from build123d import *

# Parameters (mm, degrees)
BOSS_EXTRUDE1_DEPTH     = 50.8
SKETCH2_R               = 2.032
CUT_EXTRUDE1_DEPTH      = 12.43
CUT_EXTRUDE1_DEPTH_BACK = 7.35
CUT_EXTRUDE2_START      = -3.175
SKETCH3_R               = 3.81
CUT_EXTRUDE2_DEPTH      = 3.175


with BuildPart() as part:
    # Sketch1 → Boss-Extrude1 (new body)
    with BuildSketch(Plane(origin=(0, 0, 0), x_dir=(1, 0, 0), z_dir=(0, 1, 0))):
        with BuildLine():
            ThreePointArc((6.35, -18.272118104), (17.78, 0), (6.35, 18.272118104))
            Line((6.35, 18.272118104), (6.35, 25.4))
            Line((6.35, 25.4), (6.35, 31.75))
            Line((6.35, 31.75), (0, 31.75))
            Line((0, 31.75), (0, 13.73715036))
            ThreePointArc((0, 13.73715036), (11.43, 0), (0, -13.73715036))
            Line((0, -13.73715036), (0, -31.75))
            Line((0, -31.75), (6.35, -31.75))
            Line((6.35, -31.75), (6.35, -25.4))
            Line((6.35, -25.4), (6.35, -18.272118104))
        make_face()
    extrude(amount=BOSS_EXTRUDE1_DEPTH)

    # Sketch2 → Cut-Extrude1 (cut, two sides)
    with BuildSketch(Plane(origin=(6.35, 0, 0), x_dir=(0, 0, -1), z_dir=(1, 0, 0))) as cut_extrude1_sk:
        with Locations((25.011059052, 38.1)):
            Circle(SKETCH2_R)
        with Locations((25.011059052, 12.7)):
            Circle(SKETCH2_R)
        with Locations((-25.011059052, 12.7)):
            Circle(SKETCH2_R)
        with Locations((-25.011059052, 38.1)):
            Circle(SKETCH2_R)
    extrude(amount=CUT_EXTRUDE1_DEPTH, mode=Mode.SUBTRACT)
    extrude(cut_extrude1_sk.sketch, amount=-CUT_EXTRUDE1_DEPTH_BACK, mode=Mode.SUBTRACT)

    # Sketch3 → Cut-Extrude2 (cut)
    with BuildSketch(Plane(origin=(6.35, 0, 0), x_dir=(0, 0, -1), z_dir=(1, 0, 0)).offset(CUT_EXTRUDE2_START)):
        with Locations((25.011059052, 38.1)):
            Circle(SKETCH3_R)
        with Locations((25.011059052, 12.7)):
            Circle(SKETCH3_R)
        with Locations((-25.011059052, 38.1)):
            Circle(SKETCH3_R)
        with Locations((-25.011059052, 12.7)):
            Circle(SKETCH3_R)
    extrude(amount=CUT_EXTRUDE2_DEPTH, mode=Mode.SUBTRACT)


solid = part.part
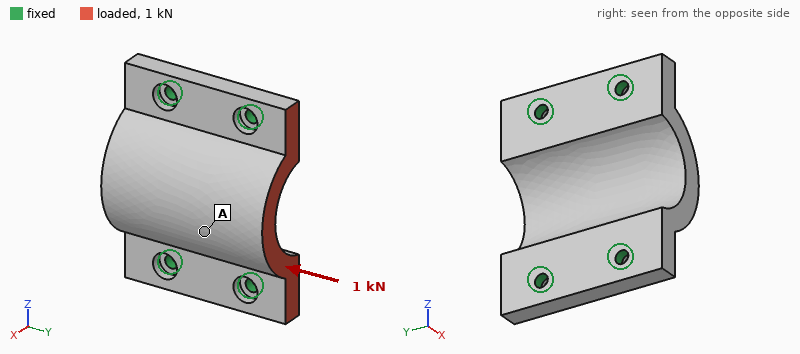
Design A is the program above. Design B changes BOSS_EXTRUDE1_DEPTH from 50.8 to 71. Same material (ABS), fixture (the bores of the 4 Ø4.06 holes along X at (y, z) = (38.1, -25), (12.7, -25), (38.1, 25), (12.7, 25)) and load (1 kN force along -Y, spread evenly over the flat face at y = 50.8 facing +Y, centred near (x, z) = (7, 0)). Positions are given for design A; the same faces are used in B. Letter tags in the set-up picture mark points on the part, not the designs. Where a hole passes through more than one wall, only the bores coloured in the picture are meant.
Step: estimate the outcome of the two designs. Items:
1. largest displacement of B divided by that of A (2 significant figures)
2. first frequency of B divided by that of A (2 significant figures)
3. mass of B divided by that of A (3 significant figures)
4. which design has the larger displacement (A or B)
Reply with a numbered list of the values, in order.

1. 1.6
2. 0.46
3. 1.41
4. B
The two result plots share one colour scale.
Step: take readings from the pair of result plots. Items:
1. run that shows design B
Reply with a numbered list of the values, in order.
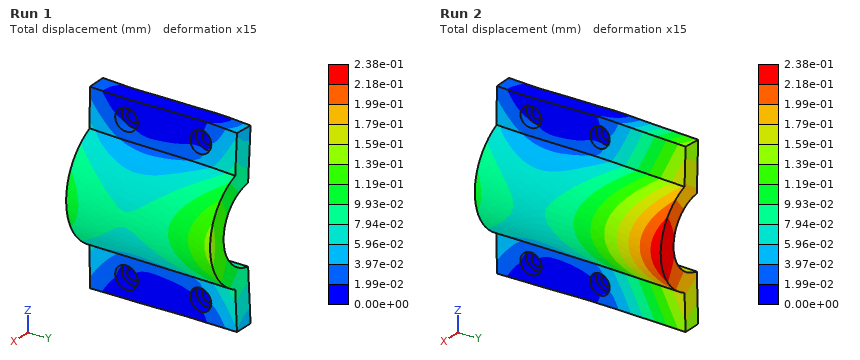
1. Run 2
